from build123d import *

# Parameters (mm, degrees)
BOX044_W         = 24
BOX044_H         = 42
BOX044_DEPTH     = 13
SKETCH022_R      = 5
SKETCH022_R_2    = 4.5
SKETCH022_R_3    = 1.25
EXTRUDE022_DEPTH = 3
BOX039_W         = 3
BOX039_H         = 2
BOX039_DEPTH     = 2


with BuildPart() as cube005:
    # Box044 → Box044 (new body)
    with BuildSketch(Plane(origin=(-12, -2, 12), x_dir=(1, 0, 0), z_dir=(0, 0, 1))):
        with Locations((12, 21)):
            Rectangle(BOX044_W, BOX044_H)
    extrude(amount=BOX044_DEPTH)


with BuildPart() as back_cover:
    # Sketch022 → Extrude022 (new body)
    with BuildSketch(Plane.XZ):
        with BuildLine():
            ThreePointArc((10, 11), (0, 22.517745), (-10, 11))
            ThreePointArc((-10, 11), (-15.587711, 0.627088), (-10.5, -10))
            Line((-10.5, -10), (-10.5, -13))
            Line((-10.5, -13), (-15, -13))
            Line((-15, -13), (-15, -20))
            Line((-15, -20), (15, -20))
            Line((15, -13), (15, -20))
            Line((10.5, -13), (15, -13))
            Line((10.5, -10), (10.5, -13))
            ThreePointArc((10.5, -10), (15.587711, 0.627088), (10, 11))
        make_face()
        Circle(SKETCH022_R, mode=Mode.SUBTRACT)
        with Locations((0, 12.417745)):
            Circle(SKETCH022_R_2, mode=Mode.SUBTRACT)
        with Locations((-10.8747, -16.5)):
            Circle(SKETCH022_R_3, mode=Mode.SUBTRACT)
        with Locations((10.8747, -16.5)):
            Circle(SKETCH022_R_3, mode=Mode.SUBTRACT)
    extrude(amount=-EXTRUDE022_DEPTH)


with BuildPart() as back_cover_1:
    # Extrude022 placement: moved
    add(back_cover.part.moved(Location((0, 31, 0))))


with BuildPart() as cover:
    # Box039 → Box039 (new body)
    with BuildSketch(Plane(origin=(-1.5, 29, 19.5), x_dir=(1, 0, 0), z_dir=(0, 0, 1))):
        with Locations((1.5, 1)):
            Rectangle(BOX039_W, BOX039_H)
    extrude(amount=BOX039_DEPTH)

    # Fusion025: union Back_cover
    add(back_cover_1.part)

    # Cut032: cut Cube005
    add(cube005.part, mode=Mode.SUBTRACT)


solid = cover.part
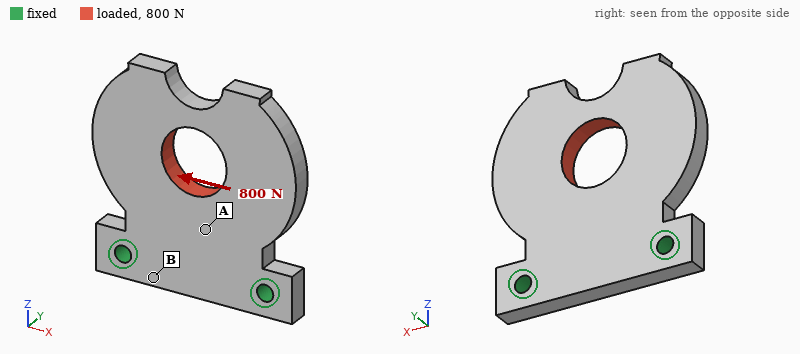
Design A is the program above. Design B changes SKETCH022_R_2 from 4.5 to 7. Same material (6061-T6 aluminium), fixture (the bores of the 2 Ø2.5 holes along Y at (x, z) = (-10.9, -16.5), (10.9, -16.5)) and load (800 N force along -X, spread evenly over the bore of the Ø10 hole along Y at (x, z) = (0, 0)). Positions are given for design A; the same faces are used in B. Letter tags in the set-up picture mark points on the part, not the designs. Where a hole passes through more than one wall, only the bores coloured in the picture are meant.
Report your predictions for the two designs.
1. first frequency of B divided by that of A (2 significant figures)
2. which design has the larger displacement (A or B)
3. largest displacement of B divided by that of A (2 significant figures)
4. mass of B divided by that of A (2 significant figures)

1.1
B
1.3
0.94
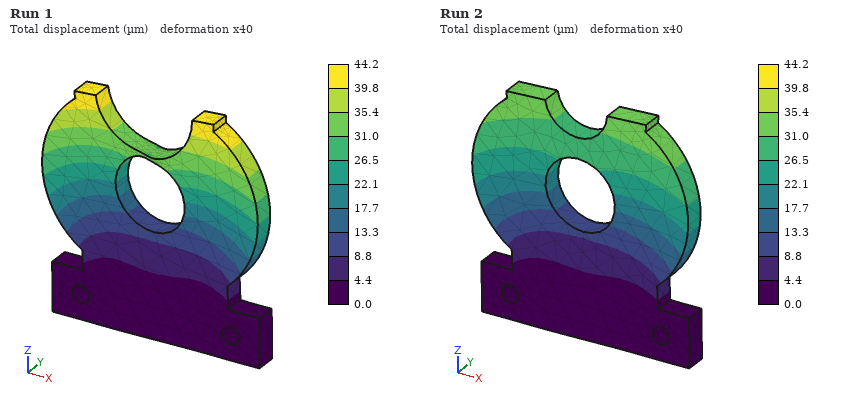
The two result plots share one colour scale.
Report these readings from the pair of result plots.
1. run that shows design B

Run 1
